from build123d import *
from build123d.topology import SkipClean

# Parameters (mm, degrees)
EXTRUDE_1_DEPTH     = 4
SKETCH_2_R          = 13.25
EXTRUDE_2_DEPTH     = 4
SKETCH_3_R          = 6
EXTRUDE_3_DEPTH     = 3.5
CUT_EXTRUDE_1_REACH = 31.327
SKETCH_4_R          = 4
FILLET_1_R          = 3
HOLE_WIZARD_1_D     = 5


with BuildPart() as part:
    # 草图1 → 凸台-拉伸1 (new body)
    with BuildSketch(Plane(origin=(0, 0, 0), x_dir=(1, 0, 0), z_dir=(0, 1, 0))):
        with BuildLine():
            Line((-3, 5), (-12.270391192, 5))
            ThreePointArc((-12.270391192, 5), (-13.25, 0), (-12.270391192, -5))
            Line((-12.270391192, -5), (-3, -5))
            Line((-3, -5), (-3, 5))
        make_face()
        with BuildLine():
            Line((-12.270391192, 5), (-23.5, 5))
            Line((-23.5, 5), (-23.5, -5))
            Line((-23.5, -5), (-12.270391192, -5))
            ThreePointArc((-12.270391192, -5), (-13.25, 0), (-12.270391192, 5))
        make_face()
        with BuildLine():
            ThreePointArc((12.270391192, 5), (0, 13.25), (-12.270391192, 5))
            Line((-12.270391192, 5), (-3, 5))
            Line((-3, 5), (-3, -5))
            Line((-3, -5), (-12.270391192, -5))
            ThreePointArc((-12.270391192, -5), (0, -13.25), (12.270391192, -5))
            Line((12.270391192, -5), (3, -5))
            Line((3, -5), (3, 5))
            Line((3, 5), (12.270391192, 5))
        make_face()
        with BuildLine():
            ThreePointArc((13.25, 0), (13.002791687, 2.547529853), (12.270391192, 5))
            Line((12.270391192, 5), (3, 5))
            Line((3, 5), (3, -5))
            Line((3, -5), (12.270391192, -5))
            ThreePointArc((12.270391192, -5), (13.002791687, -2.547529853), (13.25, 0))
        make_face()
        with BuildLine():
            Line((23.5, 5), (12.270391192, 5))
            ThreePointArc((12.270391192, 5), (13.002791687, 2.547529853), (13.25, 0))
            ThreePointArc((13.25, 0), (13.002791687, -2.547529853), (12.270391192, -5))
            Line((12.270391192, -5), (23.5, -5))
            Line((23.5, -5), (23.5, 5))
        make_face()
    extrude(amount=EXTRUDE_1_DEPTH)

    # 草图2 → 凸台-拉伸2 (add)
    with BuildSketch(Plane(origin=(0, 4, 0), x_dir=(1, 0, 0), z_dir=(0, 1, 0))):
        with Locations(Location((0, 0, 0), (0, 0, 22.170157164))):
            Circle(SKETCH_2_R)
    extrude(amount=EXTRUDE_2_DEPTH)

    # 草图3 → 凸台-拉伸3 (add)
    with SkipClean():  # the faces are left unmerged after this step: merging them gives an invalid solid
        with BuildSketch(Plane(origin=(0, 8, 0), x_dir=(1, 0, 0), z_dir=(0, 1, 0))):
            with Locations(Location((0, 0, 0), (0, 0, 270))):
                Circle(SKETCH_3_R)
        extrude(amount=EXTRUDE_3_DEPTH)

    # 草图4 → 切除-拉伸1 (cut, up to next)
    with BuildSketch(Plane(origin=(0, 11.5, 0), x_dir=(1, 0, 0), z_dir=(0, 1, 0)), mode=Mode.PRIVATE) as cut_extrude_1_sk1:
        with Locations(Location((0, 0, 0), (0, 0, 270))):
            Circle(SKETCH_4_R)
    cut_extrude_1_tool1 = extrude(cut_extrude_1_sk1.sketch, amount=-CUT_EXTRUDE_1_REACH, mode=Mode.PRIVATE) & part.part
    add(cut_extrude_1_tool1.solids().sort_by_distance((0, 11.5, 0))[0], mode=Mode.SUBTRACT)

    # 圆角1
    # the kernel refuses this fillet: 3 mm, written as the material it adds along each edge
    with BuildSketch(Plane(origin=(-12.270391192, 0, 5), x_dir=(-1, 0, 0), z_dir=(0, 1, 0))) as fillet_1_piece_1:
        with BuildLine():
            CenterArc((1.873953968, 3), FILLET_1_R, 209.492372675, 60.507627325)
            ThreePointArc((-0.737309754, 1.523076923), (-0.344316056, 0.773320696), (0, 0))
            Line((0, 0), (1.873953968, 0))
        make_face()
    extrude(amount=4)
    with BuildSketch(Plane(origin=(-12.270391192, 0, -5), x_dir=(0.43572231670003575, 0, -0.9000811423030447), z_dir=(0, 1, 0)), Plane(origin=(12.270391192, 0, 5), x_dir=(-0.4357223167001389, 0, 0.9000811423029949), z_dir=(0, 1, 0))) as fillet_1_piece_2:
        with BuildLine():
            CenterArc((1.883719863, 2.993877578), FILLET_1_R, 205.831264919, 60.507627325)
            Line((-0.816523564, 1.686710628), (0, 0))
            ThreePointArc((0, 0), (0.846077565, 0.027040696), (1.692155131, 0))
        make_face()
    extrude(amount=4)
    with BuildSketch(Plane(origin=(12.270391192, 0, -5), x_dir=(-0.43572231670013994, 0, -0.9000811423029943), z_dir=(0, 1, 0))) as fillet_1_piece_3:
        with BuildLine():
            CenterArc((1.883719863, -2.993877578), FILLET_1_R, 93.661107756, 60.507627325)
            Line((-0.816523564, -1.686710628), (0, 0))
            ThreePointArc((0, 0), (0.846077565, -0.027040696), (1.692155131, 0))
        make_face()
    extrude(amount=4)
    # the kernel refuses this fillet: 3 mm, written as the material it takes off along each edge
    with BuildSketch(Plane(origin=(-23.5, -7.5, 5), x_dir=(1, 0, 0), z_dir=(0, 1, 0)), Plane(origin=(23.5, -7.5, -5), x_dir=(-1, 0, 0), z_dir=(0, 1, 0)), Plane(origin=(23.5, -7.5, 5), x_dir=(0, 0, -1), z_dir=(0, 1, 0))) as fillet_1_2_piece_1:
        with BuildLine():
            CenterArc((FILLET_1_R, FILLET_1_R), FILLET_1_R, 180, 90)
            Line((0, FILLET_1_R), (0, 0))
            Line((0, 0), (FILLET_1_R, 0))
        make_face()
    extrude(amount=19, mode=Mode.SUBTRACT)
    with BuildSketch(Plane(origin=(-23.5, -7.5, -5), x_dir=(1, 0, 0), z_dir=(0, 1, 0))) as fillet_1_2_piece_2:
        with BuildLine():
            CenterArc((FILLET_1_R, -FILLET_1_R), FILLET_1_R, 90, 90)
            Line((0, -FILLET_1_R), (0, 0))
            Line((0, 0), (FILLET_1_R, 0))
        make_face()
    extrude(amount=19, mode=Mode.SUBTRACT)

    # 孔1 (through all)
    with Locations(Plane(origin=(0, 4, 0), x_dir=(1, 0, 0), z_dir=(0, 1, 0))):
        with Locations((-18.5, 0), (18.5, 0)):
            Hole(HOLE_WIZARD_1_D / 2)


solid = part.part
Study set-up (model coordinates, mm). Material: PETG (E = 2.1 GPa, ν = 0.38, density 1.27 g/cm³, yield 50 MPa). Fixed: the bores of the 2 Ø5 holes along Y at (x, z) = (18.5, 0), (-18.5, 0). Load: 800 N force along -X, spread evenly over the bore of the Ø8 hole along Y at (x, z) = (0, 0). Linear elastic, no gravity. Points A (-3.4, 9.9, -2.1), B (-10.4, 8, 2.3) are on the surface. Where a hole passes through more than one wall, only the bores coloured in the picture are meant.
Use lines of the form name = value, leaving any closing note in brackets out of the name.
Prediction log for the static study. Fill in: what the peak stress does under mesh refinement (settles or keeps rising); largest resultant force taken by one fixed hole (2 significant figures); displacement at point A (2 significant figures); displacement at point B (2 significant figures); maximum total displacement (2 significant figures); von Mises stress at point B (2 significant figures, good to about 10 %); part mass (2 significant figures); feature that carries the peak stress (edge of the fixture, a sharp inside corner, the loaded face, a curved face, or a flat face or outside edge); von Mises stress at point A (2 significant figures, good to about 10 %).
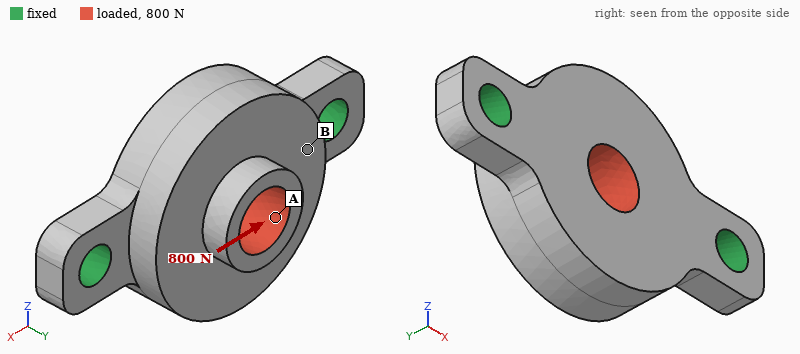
what the peak stress does under mesh refinement = keeps rising
largest resultant force taken by one fixed hole = 410 N
displacement at point A = 80 µm
displacement at point B = 48 µm
maximum total displacement = 96 µm
von Mises stress at point B = 2.7 MPa
part mass = 6.2 g
feature that carries the peak stress = edge of the fixture
von Mises stress at point A = 6.6 MPa
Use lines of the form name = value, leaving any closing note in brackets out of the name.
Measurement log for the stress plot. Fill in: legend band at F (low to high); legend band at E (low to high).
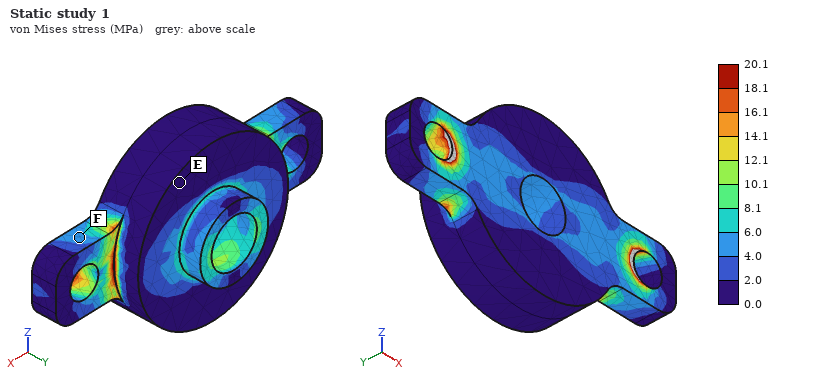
legend band at F = 4.0 to 6.0 MPa
legend band at E = 0.0 to 2.0 MPa
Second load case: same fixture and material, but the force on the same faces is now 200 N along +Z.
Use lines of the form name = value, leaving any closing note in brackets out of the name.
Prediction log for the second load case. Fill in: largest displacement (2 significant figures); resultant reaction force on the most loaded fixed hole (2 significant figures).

largest displacement = 0.20 mm
resultant reaction force on the most loaded fixed hole = 100 N
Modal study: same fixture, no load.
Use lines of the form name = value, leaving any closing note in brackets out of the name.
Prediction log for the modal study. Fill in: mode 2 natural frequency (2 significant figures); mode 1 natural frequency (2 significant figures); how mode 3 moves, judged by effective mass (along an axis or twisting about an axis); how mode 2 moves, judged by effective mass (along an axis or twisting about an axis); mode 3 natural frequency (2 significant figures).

mode 2 natural frequency = 3800 Hz
mode 1 natural frequency = 2200 Hz
how mode 3 moves, judged by effective mass = along Z
how mode 2 moves, judged by effective mass = along Y
mode 3 natural frequency = 5900 Hz
